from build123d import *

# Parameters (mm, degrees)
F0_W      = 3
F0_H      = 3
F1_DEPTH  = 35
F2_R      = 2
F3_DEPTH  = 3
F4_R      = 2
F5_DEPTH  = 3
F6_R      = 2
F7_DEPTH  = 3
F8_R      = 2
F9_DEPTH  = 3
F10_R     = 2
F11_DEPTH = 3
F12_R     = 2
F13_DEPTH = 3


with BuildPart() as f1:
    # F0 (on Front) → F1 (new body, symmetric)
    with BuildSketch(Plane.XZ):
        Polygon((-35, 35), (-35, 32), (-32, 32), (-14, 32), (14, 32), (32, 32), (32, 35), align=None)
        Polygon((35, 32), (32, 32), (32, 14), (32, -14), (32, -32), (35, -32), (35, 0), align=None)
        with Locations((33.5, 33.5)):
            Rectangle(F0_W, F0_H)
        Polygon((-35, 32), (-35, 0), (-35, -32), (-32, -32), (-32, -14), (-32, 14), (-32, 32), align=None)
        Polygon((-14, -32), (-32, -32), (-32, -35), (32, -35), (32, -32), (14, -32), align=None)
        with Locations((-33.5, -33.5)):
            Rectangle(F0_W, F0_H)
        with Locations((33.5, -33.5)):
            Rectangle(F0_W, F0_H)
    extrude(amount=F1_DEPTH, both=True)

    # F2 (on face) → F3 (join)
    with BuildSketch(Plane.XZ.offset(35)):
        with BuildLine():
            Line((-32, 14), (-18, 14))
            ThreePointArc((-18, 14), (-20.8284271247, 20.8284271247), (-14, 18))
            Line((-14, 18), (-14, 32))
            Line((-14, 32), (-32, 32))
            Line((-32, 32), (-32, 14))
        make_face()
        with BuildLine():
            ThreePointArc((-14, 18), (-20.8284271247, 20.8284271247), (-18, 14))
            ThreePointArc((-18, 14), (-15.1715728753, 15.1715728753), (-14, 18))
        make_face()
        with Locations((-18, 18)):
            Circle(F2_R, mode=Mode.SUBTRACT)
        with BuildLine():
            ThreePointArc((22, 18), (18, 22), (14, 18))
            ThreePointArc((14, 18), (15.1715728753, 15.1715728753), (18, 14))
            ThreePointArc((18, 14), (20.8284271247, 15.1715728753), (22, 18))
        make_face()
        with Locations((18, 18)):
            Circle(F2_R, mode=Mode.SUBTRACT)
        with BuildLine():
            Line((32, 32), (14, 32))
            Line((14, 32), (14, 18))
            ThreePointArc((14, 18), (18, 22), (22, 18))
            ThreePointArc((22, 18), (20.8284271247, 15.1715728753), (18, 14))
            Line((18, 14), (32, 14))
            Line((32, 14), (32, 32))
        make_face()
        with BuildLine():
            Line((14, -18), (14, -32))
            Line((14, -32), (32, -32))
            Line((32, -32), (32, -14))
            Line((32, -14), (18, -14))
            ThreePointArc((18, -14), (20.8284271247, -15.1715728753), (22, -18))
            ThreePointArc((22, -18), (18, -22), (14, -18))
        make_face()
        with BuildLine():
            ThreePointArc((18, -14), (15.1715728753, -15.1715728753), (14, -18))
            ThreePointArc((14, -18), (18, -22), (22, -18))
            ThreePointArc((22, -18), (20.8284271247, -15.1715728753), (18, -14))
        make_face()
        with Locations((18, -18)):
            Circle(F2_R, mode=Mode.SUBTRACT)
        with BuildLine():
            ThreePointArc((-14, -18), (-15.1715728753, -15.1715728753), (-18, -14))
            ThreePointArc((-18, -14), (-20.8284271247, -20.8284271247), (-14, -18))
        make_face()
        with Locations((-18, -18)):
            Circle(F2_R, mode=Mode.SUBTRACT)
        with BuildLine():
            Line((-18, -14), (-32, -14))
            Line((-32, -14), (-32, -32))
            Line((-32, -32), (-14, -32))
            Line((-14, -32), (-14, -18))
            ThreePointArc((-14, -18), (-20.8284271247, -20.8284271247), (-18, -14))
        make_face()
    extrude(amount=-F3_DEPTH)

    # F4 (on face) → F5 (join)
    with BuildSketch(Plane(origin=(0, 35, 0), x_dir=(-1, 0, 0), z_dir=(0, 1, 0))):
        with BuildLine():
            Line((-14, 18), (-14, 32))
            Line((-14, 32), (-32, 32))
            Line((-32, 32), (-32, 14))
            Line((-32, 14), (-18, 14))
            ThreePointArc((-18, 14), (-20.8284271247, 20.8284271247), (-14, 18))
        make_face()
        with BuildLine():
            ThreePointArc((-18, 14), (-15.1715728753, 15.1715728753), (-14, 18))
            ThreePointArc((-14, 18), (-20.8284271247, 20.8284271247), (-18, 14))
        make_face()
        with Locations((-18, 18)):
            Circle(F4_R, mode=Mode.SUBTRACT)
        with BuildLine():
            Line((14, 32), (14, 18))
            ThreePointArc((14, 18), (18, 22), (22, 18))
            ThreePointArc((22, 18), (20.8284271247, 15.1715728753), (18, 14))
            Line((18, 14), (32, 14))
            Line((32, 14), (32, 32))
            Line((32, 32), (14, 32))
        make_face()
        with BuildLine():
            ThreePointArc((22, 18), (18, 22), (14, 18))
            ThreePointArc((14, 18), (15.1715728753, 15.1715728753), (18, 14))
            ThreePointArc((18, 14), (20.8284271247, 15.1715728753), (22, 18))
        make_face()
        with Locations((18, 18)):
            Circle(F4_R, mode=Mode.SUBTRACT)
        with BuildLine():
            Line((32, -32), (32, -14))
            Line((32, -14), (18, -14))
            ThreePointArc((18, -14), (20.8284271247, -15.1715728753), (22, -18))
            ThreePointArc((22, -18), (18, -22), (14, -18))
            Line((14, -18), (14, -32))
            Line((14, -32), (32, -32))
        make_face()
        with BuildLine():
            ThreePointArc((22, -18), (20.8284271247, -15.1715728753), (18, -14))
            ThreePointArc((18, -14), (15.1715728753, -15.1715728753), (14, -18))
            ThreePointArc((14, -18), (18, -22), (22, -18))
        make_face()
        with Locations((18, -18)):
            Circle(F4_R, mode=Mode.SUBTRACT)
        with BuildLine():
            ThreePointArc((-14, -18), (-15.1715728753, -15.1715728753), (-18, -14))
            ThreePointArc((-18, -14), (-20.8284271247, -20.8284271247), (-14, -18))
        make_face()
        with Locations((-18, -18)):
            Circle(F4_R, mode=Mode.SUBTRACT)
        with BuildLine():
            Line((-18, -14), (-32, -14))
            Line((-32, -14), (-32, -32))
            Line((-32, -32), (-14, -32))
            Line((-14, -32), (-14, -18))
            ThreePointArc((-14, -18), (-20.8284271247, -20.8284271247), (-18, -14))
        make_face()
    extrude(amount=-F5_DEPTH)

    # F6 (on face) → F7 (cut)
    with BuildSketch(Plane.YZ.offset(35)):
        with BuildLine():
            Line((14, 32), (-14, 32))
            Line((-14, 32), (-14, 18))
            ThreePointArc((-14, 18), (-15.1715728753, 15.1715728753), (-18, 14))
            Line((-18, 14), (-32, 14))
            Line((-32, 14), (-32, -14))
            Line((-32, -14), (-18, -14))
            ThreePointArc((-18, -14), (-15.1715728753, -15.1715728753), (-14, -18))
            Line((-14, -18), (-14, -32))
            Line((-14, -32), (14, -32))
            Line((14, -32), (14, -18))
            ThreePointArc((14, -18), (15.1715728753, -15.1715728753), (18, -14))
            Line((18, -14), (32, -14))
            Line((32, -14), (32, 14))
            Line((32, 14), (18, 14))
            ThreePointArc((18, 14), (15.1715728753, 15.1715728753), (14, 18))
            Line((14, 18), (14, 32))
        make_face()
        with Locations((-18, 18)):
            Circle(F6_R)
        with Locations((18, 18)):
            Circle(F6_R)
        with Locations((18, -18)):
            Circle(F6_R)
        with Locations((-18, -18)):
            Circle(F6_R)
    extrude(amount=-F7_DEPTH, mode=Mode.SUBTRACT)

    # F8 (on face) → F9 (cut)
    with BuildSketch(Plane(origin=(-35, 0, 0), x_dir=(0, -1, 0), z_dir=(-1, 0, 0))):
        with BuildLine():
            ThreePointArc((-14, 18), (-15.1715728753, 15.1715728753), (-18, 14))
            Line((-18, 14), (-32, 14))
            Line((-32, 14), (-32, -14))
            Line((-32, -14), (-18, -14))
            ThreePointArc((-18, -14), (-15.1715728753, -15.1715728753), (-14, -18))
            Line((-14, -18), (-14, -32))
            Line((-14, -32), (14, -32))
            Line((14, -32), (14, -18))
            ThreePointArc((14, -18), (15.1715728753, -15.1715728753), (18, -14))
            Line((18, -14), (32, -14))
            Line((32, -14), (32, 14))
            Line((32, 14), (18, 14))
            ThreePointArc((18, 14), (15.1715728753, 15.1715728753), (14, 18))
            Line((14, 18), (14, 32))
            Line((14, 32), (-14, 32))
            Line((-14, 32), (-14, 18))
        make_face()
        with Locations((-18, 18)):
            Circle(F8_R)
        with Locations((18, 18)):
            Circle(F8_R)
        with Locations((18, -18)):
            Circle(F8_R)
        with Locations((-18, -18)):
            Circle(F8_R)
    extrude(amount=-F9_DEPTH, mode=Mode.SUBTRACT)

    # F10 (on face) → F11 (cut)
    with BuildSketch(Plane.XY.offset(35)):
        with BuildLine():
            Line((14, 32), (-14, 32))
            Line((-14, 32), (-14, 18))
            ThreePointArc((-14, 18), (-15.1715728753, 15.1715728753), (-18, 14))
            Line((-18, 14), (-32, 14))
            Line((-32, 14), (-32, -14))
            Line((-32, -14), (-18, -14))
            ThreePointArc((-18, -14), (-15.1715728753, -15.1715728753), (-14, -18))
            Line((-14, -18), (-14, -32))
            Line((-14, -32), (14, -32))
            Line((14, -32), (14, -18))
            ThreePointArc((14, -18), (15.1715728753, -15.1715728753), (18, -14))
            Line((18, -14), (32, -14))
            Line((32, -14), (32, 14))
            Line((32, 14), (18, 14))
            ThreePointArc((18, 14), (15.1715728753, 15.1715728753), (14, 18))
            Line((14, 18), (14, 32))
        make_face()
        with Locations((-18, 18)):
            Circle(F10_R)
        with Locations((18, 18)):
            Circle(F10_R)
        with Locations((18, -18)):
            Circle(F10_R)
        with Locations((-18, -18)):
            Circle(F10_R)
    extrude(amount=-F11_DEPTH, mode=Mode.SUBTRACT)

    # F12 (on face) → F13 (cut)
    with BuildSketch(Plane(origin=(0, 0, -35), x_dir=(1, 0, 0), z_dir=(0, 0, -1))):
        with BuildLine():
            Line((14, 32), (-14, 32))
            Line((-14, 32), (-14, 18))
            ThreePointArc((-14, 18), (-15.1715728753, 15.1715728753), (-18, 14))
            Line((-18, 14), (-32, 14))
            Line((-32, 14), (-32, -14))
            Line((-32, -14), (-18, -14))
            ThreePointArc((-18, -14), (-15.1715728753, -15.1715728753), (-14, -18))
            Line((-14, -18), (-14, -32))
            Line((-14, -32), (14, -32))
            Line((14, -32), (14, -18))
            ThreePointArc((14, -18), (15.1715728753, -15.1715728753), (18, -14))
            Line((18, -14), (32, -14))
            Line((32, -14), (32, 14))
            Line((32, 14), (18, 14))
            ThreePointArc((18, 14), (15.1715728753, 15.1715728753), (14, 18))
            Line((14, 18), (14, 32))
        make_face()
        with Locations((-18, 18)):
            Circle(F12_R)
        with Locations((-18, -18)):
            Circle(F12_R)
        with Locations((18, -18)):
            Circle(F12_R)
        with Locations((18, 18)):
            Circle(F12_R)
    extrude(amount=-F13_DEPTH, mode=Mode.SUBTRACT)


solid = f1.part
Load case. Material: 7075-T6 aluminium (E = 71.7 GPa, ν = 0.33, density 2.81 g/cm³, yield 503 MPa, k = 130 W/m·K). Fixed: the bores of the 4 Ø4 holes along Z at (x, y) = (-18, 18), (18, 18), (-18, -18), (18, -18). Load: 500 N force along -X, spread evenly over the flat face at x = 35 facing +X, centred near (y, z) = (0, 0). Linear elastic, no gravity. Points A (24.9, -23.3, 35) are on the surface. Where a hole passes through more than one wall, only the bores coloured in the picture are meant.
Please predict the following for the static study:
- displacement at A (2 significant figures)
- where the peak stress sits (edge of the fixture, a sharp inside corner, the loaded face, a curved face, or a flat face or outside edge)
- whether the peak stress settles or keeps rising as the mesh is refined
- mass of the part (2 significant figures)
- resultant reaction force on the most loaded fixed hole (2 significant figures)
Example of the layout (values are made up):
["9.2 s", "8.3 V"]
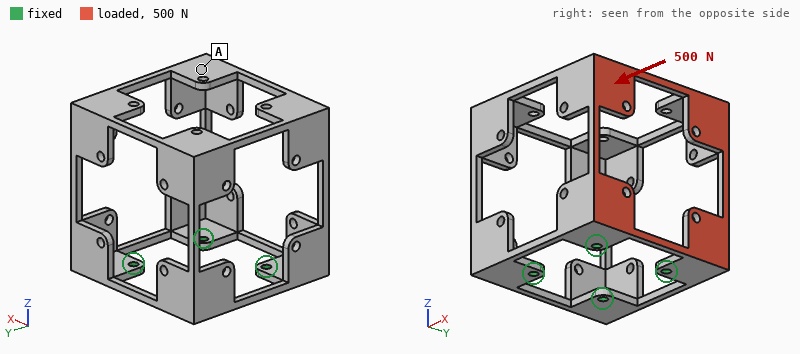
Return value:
["0.93 mm", "edge of the fixture", "keeps rising", "82 g", "210 N"]
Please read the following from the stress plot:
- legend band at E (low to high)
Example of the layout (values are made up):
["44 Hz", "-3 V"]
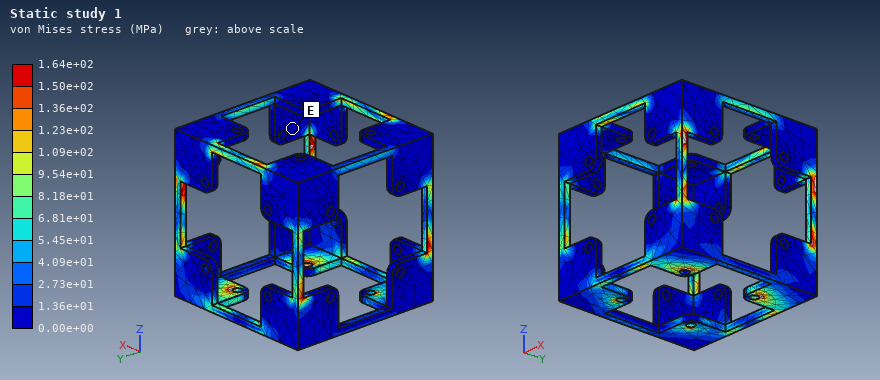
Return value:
["0.00e+00 to 1.36e+01 MPa"]
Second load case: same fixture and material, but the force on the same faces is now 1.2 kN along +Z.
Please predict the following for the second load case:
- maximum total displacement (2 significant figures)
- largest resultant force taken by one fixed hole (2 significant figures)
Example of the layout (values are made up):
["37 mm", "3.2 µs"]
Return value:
["1.3 mm", "650 N"]
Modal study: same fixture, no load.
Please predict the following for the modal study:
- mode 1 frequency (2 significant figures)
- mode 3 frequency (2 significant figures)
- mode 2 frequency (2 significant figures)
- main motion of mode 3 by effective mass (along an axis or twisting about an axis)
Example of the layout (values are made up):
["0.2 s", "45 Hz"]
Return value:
["450 Hz", "690 Hz", "450 Hz", "twisting about Z"]
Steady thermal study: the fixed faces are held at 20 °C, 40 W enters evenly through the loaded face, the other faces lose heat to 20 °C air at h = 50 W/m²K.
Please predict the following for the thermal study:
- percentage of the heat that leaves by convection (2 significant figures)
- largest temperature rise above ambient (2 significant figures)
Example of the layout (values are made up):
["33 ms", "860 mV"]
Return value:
["54 %", "63 K"]
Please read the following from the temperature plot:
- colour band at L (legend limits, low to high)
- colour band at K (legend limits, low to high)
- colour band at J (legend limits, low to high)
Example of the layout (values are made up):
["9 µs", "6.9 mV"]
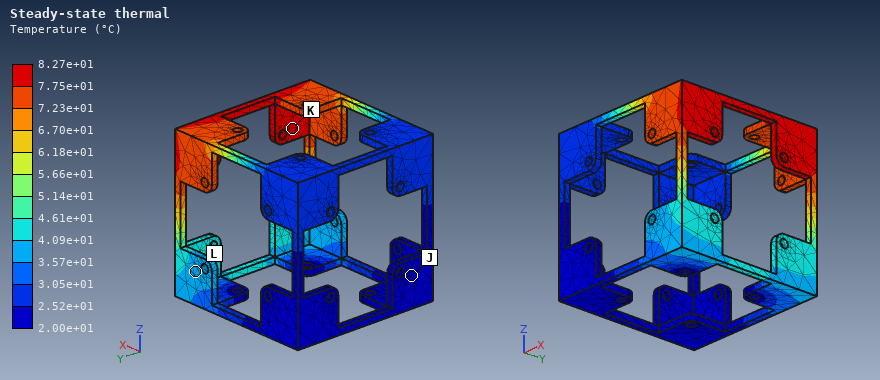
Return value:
["3.57e+01 to 4.09e+01 °C", "7.75e+01 to 8.27e+01 °C", "2.00e+01 to 2.52e+01 °C"]
